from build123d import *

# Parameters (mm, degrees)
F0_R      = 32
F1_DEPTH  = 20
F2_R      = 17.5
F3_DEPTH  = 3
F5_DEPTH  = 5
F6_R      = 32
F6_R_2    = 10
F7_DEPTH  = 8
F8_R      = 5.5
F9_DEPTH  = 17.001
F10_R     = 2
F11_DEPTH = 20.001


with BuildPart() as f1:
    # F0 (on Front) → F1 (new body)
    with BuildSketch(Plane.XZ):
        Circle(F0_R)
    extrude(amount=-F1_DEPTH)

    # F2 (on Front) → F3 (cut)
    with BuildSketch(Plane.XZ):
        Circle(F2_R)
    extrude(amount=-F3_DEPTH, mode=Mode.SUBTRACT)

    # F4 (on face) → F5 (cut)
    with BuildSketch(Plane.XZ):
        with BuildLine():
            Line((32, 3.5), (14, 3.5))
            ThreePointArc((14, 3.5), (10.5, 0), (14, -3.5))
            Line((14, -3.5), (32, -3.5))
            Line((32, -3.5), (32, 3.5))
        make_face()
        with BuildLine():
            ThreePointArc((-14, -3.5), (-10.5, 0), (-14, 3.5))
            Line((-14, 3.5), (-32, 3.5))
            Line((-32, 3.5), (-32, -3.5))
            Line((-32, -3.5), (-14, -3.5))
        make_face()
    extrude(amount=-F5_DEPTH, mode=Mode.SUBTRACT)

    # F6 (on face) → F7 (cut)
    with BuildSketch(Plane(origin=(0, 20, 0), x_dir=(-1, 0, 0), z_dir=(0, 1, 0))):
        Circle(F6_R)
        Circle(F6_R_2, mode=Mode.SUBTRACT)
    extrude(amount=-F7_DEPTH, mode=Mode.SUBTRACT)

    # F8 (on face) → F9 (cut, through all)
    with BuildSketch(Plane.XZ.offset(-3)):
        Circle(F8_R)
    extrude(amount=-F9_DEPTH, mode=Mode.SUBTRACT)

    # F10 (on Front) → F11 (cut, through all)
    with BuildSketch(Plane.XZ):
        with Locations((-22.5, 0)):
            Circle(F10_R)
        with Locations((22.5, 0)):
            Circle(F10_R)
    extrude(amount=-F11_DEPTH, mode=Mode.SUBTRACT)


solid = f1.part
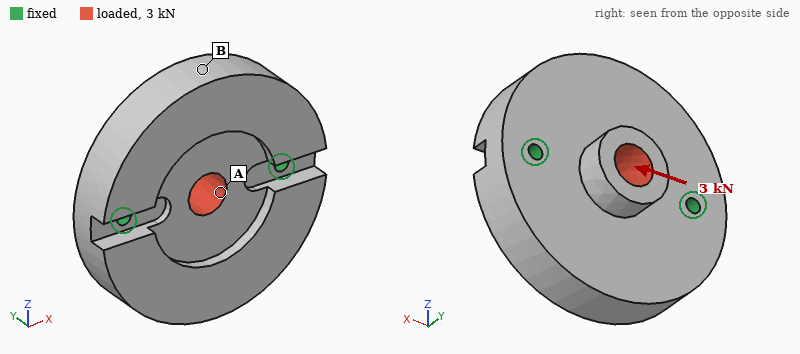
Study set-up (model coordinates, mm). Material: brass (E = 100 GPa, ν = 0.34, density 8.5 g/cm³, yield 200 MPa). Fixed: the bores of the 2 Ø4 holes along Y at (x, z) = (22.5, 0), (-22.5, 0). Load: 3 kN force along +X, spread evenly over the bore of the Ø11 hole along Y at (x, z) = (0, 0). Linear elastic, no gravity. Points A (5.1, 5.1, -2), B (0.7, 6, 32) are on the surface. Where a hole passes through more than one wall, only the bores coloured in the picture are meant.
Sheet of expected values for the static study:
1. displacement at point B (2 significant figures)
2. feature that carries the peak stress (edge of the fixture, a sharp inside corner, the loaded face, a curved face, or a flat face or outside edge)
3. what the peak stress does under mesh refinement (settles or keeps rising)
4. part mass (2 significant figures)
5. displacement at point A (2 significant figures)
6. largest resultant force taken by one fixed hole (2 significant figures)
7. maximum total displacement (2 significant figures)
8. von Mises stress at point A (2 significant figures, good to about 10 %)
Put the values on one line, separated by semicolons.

1.2 µm; edge of the fixture; keeps rising; 300 g; 1.9 µm; 1.5 kN; 5.0 µm; 7.2 MPa
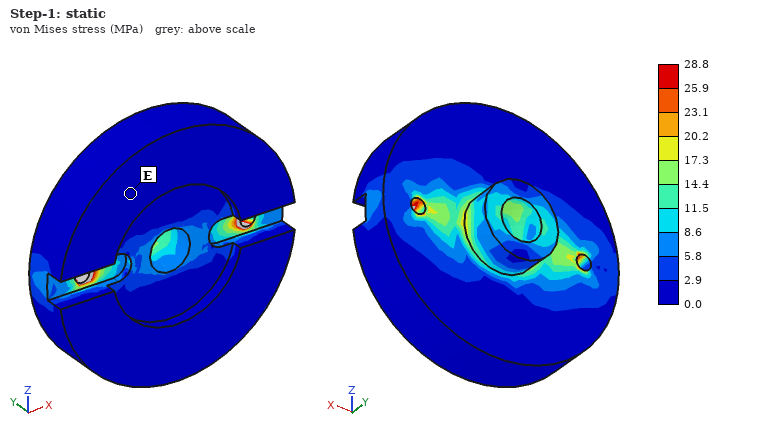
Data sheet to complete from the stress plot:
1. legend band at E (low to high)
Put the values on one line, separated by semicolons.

0.0 to 2.9 MPa
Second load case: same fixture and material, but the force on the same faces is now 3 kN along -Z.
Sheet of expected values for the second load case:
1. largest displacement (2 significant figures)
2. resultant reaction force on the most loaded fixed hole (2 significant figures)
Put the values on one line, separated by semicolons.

12 µm; 1.5 kN
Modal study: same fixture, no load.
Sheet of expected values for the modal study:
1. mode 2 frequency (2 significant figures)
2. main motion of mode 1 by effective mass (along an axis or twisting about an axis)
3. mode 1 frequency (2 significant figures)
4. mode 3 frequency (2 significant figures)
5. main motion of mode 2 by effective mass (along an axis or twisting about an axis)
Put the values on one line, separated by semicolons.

4400 Hz; twisting about X; 2800 Hz; 9100 Hz; along Y
